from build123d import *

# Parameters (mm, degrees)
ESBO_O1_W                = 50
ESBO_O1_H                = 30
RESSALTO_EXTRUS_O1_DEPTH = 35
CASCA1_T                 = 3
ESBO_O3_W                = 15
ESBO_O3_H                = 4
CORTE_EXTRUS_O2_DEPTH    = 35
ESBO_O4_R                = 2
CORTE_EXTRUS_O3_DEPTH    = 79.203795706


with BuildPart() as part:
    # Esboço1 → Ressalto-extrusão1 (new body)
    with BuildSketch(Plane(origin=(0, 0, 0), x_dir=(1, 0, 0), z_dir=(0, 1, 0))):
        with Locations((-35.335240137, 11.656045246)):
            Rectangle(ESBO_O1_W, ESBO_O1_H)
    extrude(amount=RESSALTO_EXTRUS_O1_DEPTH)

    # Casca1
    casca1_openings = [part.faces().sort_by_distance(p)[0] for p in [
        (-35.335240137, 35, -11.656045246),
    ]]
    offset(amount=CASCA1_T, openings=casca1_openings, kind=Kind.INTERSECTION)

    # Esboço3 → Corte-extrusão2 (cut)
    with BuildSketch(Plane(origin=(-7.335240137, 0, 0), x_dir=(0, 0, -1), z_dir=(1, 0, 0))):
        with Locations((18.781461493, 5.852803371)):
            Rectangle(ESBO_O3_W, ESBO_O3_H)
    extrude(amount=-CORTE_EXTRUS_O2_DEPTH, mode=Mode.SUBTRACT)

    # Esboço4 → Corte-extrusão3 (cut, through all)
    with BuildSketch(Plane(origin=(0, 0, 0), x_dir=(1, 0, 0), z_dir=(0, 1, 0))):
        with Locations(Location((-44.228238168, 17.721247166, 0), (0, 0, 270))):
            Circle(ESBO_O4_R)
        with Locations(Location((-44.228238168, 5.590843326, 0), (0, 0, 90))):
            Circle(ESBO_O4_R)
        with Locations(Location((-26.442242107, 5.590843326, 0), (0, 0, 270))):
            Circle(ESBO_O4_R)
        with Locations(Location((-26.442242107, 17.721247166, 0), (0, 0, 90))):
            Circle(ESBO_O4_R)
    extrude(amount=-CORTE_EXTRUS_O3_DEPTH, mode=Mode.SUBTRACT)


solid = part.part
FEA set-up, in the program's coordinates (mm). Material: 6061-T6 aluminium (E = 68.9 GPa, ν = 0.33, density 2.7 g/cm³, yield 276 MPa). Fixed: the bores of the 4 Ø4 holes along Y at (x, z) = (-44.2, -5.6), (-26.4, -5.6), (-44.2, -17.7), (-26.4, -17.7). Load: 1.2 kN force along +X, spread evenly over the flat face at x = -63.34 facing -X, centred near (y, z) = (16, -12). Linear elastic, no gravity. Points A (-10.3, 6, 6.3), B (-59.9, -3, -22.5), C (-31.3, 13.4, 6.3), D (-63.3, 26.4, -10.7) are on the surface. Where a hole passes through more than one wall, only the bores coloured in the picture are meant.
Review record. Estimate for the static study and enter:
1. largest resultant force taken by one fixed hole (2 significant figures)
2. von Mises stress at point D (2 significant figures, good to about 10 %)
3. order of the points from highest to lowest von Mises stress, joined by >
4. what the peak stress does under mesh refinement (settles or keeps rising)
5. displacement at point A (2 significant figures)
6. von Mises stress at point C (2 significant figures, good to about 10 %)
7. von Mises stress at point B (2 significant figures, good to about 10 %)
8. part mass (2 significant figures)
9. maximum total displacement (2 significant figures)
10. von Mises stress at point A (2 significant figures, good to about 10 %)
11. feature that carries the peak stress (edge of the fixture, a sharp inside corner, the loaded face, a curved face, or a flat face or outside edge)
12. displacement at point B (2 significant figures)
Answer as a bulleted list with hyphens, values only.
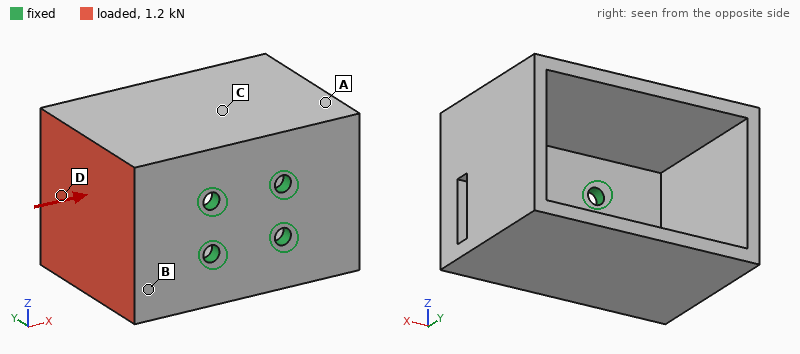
- 570 N
- 36 MPa
- D > B > C > A
- keeps rising
- 0.047 mm
- 14 MPa
- 24 MPa
- 64 g
- 0.13 mm
- 7.1 MPa
- edge of the fixture
- 0.041 mm
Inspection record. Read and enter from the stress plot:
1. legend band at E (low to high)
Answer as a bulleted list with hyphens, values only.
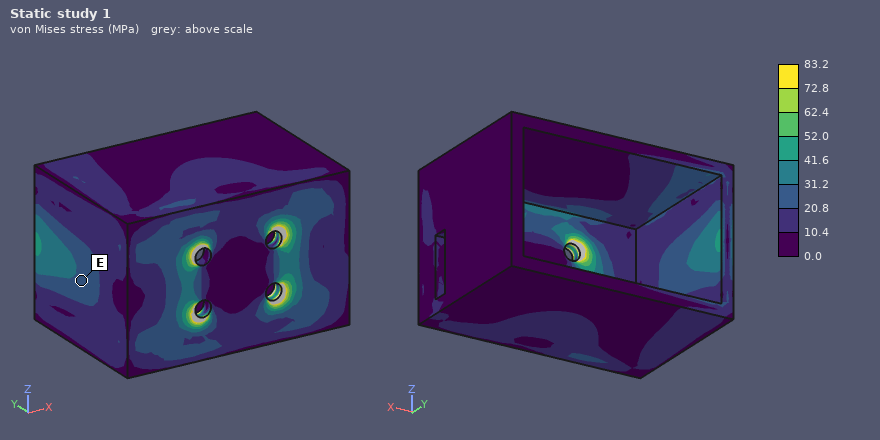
- 20.8 to 31.2 MPa
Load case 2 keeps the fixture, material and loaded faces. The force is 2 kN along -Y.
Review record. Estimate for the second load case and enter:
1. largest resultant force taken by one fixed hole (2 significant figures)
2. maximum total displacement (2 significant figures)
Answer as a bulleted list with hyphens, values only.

- 1.6 kN
- 0.24 mm
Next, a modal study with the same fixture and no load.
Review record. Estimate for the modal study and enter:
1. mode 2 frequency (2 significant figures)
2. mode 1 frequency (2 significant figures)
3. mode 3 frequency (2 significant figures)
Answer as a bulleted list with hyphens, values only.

- 2600 Hz
- 2500 Hz
- 2900 Hz
